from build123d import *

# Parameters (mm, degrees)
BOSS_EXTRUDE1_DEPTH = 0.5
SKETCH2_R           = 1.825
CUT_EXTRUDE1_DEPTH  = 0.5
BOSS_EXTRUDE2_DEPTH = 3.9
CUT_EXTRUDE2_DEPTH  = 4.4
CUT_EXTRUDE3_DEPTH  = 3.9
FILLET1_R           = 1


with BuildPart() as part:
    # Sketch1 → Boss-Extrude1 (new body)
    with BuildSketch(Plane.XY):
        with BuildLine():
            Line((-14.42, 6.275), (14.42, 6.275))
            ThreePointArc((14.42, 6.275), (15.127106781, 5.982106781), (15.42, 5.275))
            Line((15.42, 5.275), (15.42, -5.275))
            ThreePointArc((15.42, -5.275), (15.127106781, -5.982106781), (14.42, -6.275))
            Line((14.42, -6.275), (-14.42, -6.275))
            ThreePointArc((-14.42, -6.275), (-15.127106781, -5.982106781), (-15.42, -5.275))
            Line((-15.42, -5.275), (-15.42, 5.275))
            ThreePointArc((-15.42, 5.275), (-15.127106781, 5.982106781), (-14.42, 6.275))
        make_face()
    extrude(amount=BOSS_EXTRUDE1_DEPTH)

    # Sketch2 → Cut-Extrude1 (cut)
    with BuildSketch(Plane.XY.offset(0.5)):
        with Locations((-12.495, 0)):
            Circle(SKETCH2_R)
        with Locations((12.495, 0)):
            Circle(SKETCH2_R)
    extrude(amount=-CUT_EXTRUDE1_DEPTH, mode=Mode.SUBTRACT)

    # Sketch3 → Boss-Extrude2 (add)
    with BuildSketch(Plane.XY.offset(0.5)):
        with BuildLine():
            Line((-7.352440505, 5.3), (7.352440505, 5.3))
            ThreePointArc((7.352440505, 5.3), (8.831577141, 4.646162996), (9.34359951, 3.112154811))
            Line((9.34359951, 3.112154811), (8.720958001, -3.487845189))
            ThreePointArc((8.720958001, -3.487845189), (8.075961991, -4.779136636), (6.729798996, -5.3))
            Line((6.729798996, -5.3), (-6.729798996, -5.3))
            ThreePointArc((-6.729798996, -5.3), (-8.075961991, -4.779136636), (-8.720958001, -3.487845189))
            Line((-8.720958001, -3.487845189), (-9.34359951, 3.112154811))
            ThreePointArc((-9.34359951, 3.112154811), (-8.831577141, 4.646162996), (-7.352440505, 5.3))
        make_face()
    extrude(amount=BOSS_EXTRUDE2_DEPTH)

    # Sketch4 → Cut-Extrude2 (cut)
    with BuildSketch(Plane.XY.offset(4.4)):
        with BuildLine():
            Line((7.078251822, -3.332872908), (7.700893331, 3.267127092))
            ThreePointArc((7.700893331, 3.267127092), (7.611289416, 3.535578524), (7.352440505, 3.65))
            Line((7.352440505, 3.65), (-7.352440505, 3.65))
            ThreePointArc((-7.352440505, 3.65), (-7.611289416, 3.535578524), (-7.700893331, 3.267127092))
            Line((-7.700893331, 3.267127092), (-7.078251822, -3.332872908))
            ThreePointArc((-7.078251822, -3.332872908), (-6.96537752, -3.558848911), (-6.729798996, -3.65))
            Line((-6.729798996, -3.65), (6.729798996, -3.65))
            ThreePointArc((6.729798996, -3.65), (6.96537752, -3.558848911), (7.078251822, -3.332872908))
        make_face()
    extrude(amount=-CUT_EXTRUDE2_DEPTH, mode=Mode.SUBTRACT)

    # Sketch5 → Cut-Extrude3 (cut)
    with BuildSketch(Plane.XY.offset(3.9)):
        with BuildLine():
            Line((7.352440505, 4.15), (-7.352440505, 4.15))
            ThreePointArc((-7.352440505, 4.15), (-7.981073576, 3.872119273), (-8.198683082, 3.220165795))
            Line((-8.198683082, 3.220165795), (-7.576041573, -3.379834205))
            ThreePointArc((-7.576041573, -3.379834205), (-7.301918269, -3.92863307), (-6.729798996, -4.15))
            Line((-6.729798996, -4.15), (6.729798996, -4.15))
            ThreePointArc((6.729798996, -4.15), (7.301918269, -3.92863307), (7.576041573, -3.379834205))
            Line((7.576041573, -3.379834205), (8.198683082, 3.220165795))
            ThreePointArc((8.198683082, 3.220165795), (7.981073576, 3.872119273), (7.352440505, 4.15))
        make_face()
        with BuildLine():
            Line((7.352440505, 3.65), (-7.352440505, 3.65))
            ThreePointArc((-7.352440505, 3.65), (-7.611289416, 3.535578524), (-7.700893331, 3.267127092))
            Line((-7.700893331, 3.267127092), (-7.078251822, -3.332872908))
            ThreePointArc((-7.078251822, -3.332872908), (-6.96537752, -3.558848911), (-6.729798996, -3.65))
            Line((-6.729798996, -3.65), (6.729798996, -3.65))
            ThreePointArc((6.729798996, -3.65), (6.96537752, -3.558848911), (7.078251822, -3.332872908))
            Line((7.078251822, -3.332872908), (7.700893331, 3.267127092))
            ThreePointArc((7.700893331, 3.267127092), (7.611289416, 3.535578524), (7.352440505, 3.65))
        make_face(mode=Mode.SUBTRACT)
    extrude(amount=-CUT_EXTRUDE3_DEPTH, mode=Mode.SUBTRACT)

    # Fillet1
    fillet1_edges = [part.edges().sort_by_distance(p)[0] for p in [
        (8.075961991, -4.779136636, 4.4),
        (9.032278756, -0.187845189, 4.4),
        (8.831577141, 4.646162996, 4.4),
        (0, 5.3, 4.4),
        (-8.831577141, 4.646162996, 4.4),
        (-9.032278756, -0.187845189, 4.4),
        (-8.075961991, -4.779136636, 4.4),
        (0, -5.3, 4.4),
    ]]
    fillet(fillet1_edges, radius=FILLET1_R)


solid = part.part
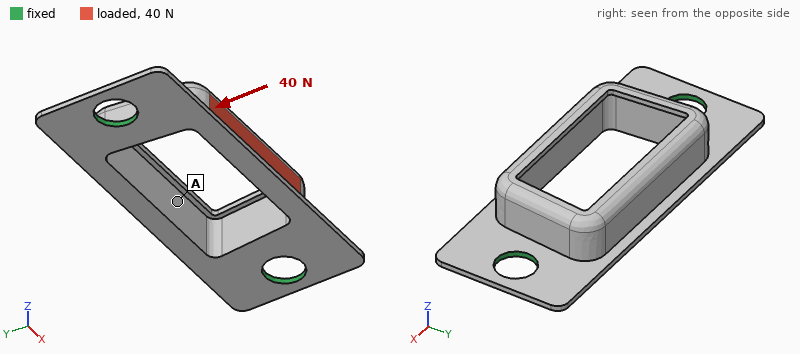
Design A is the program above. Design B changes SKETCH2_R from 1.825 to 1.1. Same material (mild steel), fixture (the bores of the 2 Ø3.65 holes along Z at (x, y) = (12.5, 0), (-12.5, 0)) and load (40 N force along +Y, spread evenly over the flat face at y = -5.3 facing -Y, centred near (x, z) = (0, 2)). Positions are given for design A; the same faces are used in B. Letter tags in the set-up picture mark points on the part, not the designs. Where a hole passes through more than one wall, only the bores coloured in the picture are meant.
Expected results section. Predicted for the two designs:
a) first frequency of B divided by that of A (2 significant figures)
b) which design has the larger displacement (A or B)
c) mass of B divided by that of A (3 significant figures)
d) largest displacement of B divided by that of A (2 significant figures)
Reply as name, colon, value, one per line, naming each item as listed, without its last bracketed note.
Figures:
first frequency of B divided by that of A: 0.70
which design has the larger displacement: B
mass of B divided by that of A: 1.02
largest displacement of B divided by that of A: 1.6
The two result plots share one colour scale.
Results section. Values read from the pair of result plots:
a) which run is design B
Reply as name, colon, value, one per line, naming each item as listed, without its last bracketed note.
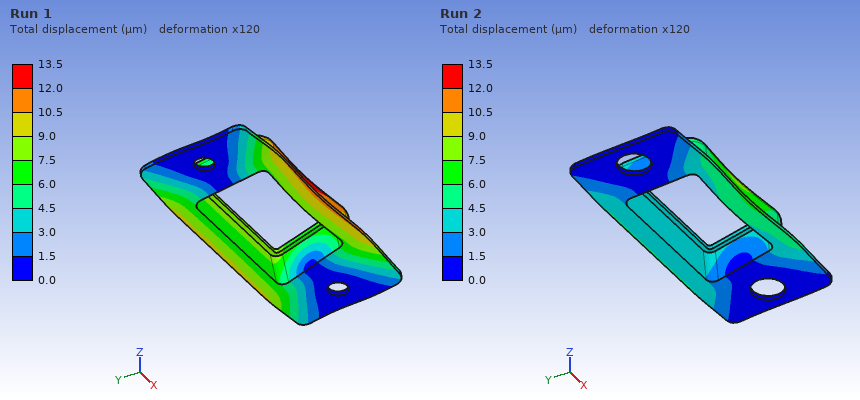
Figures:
which run is design B: Run 1
